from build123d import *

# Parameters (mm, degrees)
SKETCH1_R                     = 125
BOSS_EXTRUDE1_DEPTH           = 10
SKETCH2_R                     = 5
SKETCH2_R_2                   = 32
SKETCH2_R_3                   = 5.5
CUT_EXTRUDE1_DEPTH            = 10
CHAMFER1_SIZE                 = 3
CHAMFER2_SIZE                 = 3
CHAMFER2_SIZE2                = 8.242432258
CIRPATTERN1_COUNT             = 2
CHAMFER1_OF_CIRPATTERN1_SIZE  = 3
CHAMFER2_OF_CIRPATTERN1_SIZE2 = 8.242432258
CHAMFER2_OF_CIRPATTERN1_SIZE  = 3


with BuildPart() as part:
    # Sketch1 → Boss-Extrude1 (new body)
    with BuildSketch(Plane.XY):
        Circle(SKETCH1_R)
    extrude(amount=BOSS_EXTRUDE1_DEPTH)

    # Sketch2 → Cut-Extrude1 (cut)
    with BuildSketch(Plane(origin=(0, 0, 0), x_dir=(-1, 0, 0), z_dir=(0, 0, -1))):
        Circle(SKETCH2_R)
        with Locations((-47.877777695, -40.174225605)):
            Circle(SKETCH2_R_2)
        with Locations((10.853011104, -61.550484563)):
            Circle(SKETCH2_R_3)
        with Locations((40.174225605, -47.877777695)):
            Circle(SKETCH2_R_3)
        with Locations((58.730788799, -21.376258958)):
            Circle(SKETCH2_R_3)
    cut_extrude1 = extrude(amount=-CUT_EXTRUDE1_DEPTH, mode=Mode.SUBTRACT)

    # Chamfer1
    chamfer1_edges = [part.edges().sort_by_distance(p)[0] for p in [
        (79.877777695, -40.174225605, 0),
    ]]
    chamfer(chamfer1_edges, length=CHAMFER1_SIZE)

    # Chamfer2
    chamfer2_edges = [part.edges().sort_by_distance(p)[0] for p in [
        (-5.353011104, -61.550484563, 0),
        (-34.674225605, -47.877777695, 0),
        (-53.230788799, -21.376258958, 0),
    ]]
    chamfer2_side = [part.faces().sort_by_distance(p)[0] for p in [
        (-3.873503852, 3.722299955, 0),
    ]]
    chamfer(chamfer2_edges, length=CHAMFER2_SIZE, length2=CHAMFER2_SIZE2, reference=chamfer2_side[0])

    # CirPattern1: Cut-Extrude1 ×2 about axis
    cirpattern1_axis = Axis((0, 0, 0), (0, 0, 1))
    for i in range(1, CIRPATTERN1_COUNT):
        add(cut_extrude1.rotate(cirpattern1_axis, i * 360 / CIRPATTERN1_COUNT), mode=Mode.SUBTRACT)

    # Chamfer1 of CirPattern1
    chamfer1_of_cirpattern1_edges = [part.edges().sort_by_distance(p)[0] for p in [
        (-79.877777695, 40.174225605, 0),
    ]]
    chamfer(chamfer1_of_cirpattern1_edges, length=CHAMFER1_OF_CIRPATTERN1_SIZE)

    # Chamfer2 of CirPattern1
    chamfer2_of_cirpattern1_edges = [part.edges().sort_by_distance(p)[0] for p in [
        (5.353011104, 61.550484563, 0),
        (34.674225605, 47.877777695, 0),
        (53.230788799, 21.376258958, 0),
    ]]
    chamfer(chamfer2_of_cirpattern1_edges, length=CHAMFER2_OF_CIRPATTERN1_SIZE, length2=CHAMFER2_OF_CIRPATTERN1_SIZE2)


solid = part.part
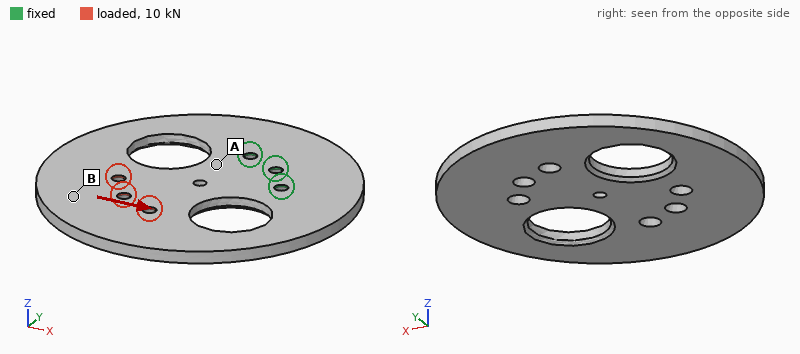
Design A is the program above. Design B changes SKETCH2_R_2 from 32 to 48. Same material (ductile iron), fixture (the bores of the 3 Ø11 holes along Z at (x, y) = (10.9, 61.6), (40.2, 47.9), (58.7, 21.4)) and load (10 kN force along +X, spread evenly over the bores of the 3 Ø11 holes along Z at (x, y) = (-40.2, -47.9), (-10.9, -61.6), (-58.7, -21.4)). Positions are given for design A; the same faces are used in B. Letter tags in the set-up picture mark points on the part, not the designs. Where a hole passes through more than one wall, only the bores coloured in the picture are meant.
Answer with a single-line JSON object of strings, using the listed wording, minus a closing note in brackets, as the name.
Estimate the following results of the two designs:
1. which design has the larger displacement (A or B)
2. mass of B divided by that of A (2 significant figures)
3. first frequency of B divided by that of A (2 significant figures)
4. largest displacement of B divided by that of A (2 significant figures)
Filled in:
{"which design has the larger displacement": "B", "mass of B divided by that of A": "0.80", "first frequency of B divided by that of A": "0.79", "largest displacement of B divided by that of A": "1.9"}
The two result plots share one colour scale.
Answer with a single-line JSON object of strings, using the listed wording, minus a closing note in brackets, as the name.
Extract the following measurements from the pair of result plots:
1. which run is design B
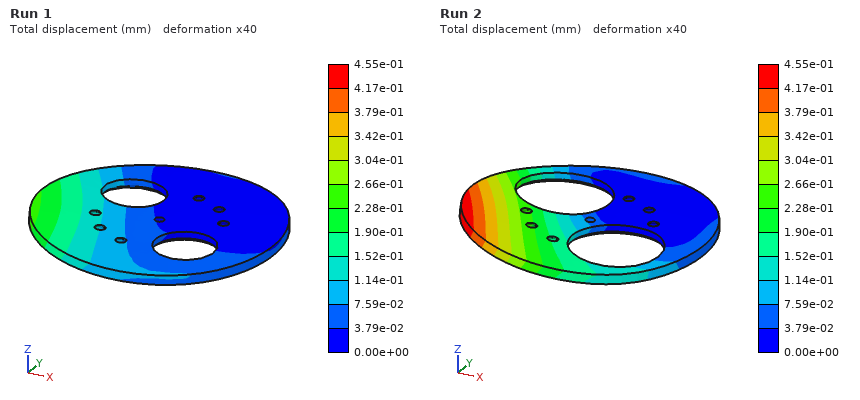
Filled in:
{"which run is design B": "Run 2"}
